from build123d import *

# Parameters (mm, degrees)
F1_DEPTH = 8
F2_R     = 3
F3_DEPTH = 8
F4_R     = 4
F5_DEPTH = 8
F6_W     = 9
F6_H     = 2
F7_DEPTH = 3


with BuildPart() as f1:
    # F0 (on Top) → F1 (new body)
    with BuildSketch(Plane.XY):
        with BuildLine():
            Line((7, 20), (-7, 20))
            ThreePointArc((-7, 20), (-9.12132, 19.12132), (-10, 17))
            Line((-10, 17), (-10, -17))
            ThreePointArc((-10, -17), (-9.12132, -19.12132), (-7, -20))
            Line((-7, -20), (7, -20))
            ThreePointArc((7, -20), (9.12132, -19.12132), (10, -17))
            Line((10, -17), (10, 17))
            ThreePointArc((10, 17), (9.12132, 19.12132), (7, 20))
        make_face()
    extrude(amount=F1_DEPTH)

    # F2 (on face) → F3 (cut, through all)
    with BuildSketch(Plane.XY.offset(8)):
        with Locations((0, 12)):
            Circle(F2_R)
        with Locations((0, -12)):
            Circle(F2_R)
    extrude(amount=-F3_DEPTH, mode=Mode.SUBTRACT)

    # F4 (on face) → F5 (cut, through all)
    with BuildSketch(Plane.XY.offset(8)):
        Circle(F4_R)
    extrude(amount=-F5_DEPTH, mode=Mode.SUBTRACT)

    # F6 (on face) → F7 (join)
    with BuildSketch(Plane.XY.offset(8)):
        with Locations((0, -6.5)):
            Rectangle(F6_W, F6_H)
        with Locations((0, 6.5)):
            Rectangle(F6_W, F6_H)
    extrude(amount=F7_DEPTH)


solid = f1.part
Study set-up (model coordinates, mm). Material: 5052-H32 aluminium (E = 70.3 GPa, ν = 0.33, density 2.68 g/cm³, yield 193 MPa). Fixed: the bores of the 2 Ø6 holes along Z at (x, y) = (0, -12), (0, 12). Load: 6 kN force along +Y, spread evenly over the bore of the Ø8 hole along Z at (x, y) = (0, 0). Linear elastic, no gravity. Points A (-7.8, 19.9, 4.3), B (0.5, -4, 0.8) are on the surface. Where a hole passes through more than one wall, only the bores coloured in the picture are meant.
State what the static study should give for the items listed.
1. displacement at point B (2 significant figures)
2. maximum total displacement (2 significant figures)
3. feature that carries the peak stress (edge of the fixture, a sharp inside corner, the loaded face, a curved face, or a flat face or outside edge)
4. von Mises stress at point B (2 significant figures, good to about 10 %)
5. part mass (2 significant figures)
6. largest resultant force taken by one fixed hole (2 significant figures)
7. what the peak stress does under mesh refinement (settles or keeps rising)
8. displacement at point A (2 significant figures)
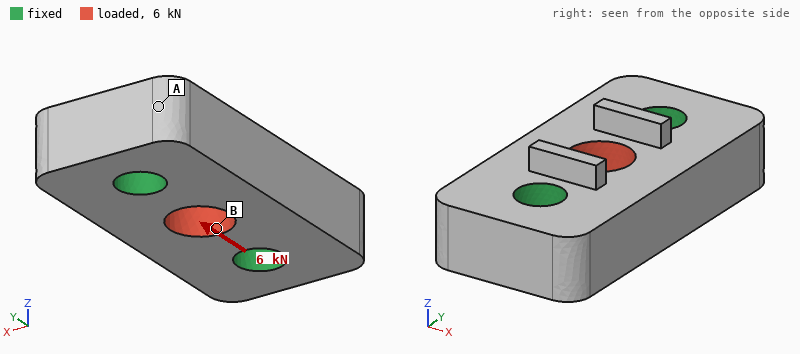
2.8 µm
4.5 µm
edge of the fixture
38 MPa
15 g
3.0 kN
keeps rising
1.4 µm
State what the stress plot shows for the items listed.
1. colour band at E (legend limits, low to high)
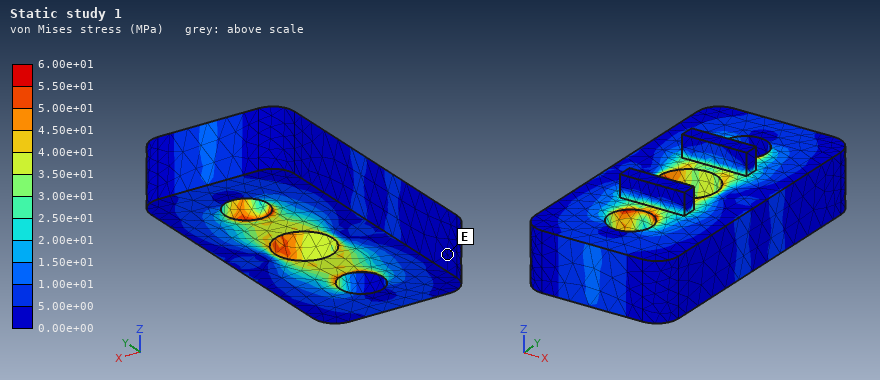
0.00e+00 to 5.00e+00 MPa
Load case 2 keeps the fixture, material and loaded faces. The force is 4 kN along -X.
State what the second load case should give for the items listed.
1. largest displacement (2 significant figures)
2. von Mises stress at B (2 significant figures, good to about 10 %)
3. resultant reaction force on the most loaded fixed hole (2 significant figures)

6.5 µm
36 MPa
2.0 kN
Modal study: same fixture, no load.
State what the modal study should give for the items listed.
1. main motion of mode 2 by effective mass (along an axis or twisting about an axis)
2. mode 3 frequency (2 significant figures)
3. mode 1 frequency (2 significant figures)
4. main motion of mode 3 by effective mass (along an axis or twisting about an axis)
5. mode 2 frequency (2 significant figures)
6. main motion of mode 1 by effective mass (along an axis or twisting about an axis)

along Z
59 kHz
44 kHz
twisting about Z
47 kHz
twisting about Y
